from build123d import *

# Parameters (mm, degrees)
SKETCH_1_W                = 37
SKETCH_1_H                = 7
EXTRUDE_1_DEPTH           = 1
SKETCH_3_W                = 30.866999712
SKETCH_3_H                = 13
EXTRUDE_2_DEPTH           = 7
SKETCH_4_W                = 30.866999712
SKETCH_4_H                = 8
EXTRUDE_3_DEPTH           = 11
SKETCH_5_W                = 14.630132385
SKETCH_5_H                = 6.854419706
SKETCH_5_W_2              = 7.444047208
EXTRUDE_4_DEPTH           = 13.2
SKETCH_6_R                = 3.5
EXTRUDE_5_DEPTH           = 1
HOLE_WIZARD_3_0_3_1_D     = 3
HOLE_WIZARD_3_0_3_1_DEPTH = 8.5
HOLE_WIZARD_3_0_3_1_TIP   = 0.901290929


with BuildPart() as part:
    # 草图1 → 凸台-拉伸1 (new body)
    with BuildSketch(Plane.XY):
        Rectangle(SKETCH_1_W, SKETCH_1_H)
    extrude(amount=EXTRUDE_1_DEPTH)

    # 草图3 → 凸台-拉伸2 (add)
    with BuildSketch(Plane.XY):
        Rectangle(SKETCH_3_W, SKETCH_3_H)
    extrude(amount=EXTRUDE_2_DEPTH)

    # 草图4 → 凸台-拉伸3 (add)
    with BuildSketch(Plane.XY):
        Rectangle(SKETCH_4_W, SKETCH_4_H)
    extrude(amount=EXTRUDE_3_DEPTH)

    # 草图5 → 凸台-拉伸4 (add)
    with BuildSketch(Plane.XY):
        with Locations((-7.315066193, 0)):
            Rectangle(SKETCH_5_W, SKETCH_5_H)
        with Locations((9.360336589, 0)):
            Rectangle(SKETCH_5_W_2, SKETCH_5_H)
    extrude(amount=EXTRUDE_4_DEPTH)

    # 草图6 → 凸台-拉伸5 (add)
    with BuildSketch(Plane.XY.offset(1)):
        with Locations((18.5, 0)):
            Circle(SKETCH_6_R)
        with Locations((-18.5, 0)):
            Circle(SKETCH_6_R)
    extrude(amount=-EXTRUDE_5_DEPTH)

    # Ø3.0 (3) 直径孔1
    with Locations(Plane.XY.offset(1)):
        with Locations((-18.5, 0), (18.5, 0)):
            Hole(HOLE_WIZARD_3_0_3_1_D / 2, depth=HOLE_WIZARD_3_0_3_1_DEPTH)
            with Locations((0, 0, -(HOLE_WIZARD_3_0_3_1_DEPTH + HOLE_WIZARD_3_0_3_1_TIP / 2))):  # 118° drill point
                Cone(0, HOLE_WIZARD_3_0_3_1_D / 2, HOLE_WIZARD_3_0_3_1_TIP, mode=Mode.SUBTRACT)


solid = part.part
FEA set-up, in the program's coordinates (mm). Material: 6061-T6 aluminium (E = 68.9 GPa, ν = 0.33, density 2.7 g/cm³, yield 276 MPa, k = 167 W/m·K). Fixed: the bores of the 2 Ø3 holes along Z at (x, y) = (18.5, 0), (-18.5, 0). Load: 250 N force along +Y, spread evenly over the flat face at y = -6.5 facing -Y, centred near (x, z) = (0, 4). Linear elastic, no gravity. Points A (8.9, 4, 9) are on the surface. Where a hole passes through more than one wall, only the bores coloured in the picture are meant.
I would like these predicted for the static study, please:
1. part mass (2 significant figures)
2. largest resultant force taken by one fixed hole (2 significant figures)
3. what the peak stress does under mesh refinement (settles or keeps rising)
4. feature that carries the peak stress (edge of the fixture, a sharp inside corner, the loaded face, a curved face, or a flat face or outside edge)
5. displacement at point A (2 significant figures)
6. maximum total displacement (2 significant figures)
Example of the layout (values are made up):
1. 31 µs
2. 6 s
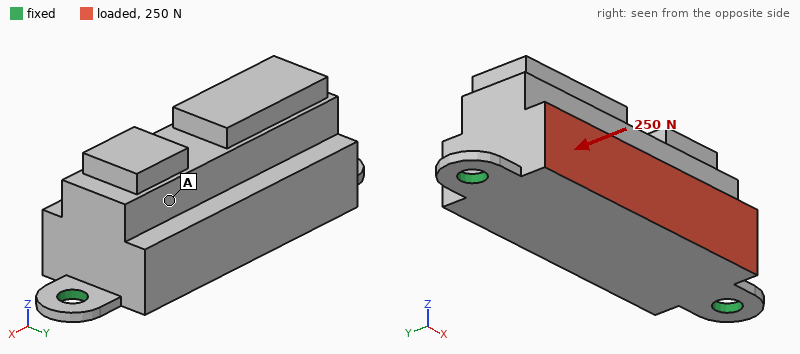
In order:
1. 11 g
2. 130 N
3. keeps rising
4. edge of the fixture
5. 65 µm
6. 90 µm
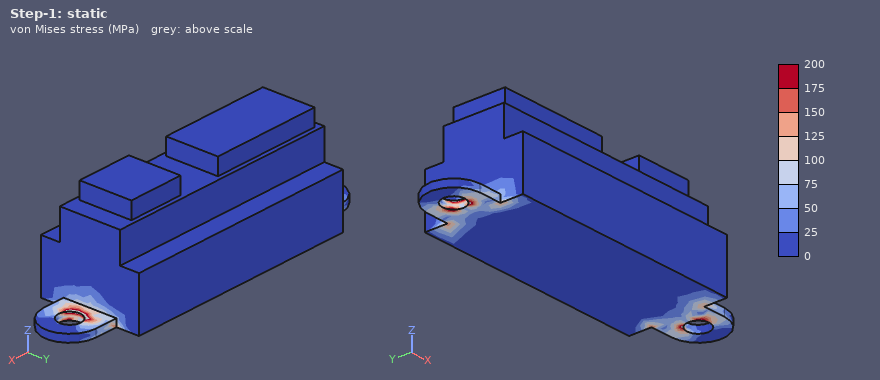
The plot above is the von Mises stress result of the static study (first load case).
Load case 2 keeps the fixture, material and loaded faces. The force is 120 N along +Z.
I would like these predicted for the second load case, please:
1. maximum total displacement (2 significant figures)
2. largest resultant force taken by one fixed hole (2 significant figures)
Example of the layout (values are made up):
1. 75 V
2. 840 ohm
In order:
1. 90 µm
2. 74 N
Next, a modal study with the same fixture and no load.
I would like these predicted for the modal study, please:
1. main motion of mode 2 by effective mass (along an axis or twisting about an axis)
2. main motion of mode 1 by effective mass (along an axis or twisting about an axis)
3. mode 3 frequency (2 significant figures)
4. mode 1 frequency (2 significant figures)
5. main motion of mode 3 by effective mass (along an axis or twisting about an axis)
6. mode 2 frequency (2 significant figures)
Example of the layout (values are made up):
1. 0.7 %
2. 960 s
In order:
1. along Z
2. along Y
3. 14 kHz
4. 2300 Hz
5. along X
6. 9000 Hz
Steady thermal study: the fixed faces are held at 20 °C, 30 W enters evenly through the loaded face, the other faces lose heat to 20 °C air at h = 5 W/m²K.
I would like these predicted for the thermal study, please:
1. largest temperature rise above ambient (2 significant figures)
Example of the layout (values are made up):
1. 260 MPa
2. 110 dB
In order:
1. 51 K
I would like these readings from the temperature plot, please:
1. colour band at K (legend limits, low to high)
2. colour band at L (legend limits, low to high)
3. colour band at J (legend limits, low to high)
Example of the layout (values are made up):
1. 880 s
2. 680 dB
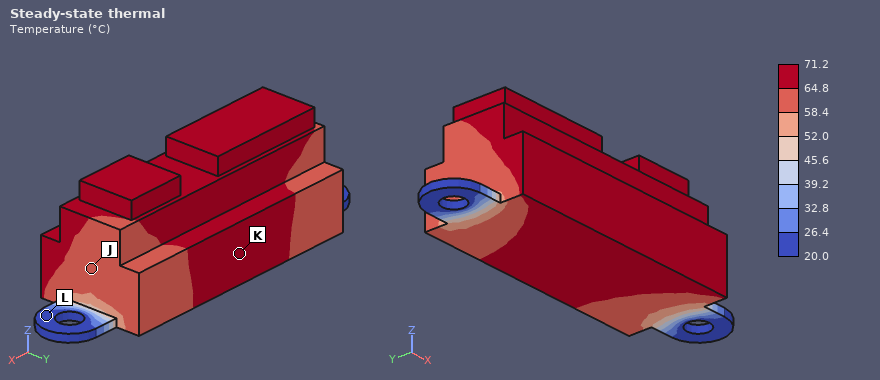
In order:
1. 64.8 to 71.2 °C
2. 20.0 to 26.4 °C
3. 58.4 to 64.8 °C
